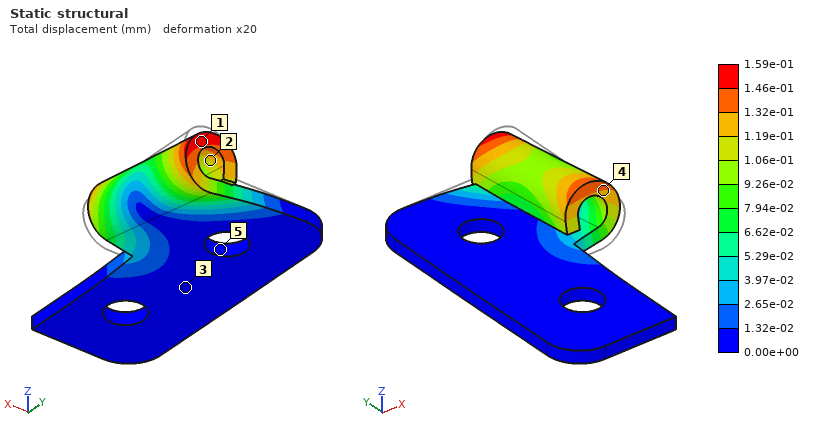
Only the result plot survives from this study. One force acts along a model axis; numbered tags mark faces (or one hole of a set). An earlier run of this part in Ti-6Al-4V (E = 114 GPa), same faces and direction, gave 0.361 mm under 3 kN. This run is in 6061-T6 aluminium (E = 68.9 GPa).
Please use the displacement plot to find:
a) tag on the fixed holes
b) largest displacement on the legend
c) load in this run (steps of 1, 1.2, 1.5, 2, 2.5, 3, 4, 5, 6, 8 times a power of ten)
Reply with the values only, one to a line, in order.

5
1.59e-01 mm
800 N
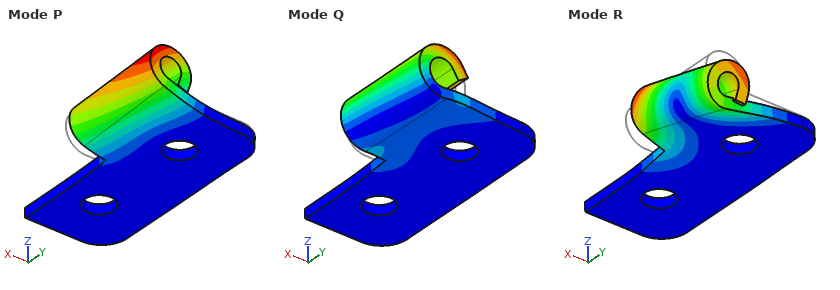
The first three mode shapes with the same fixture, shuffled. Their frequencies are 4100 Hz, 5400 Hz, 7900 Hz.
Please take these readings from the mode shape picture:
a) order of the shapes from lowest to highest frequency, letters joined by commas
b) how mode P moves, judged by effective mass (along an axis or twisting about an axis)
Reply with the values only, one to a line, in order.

P, R, Q
along Z
